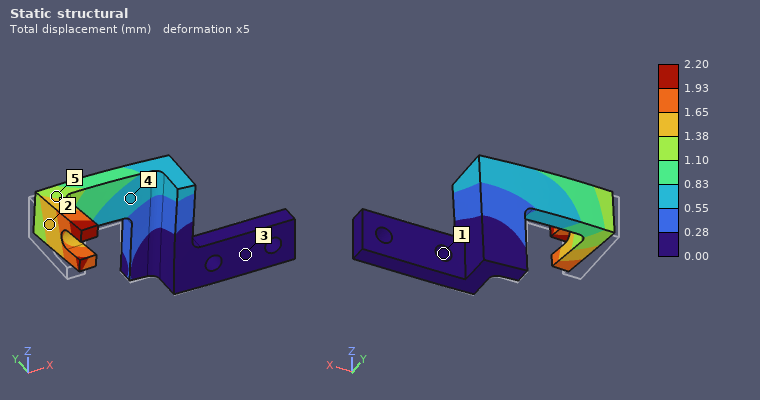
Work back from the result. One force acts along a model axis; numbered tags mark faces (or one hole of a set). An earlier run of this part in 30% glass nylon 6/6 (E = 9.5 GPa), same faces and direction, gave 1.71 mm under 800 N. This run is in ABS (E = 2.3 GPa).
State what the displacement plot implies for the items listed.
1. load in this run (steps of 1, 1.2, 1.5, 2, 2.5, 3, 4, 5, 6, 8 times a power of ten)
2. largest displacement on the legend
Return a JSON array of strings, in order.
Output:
["250 N", "2.20 mm"]
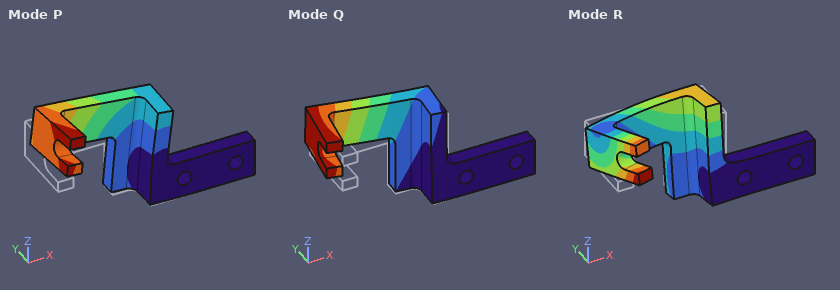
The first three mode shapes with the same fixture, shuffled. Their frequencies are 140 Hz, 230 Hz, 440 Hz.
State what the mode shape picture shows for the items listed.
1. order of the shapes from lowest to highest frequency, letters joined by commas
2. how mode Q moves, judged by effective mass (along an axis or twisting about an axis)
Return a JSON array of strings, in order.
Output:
["Q, P, R", "along Y"]
